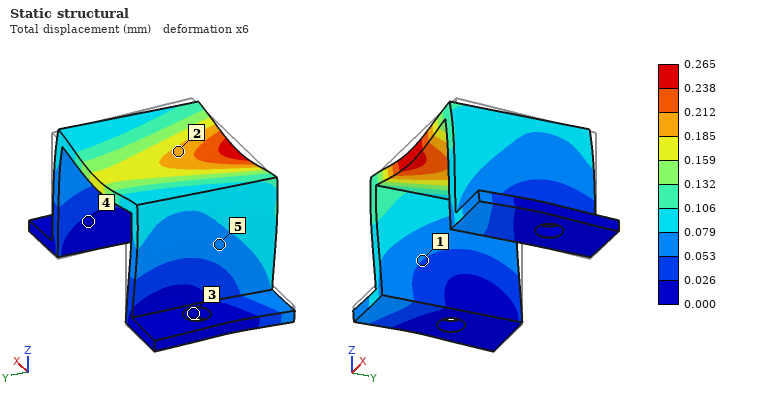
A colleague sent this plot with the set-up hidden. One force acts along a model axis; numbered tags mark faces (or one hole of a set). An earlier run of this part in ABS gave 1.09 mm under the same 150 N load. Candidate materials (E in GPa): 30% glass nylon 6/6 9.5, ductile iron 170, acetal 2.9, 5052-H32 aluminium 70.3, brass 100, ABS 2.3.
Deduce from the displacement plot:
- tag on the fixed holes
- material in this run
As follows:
3
30% glass nylon 6/6
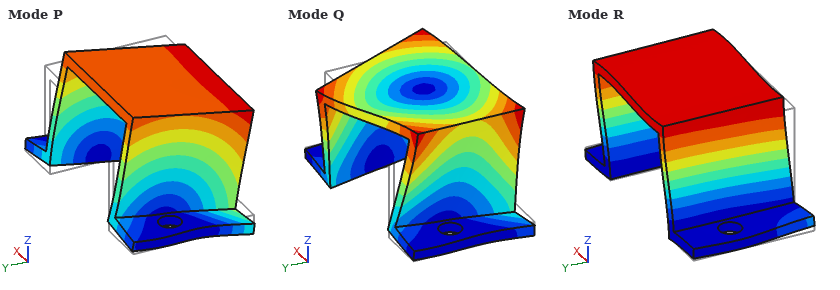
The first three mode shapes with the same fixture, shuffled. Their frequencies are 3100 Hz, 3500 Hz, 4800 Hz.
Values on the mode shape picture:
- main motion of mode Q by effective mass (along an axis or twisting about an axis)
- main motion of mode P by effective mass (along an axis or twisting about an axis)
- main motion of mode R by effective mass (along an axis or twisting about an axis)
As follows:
twisting about Z
along Y
along X
